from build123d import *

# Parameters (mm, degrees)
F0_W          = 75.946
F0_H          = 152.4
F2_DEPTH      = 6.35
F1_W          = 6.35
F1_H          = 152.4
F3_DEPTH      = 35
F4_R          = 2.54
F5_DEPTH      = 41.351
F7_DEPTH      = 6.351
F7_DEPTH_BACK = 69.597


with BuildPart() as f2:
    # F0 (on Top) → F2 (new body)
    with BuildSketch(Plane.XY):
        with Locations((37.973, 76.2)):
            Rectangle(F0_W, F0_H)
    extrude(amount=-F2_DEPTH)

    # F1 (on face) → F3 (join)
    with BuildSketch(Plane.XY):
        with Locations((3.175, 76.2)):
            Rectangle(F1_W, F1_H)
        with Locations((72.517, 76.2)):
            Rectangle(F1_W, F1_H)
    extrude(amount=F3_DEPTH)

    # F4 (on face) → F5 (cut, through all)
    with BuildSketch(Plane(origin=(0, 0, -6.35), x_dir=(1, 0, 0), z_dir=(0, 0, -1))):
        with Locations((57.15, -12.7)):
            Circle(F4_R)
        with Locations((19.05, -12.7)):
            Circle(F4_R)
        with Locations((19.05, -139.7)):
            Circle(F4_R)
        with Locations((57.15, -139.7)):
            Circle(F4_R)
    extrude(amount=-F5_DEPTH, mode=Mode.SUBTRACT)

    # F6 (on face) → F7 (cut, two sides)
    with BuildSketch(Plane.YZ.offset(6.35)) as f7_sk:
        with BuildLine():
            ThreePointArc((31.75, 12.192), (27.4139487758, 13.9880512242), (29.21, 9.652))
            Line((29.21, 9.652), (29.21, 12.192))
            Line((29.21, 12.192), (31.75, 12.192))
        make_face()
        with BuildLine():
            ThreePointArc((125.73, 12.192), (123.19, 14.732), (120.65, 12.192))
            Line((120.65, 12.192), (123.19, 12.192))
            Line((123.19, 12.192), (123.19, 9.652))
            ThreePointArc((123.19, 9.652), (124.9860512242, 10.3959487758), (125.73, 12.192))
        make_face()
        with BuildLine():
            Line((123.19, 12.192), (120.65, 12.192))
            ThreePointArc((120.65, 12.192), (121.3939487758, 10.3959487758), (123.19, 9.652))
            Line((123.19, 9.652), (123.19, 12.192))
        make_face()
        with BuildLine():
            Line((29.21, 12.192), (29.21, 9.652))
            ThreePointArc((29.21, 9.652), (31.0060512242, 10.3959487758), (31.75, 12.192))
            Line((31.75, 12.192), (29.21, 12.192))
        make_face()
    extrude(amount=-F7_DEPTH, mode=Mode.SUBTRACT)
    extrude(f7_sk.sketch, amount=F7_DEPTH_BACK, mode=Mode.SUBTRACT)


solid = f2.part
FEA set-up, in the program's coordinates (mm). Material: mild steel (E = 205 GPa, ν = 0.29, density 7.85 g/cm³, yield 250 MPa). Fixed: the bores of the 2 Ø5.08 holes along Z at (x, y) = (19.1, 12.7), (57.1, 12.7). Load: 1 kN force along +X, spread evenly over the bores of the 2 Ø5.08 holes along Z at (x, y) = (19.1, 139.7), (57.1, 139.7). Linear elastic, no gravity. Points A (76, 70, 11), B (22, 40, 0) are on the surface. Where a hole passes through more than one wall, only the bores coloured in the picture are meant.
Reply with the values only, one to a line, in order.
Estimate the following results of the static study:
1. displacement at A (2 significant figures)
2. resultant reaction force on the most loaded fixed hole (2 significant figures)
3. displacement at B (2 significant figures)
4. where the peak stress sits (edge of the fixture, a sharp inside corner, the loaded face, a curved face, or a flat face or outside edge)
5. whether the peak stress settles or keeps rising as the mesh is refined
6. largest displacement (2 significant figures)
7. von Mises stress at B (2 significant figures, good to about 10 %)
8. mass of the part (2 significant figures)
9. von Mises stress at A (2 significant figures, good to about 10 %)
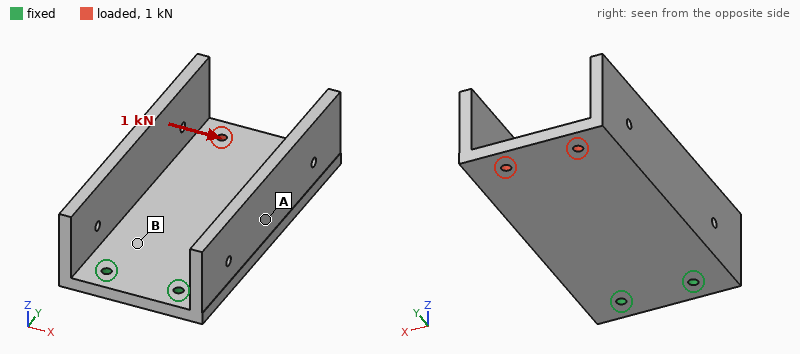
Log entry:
11 µm
3.1 kN
4.2 µm
edge of the fixture
keeps rising
27 µm
8.5 MPa
1.1 kg
3.8 MPa
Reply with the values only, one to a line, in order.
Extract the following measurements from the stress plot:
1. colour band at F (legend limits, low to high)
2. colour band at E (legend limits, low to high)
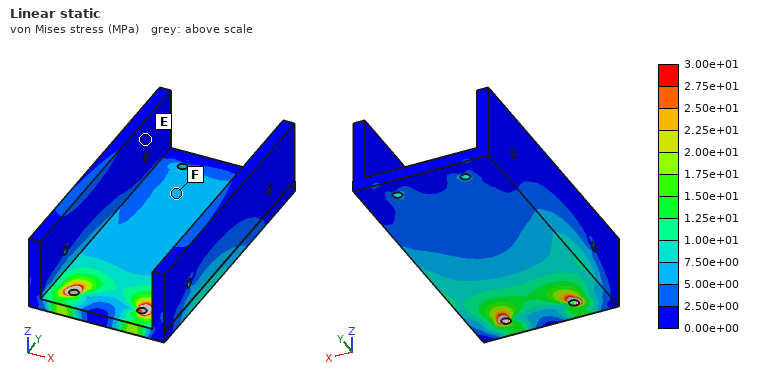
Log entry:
5.00e+00 to 7.50e+00 MPa
0.00e+00 to 2.50e+00 MPa
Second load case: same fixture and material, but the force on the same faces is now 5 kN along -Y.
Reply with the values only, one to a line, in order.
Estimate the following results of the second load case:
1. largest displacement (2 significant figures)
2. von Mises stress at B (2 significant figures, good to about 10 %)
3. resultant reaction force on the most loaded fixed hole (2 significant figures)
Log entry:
14 µm
9.8 MPa
2.5 kN
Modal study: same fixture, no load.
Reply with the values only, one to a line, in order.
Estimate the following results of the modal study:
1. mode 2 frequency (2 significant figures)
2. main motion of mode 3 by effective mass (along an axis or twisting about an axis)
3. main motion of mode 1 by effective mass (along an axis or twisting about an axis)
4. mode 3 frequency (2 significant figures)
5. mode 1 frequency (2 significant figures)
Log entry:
650 Hz
along X
along Z
1600 Hz
350 Hz
